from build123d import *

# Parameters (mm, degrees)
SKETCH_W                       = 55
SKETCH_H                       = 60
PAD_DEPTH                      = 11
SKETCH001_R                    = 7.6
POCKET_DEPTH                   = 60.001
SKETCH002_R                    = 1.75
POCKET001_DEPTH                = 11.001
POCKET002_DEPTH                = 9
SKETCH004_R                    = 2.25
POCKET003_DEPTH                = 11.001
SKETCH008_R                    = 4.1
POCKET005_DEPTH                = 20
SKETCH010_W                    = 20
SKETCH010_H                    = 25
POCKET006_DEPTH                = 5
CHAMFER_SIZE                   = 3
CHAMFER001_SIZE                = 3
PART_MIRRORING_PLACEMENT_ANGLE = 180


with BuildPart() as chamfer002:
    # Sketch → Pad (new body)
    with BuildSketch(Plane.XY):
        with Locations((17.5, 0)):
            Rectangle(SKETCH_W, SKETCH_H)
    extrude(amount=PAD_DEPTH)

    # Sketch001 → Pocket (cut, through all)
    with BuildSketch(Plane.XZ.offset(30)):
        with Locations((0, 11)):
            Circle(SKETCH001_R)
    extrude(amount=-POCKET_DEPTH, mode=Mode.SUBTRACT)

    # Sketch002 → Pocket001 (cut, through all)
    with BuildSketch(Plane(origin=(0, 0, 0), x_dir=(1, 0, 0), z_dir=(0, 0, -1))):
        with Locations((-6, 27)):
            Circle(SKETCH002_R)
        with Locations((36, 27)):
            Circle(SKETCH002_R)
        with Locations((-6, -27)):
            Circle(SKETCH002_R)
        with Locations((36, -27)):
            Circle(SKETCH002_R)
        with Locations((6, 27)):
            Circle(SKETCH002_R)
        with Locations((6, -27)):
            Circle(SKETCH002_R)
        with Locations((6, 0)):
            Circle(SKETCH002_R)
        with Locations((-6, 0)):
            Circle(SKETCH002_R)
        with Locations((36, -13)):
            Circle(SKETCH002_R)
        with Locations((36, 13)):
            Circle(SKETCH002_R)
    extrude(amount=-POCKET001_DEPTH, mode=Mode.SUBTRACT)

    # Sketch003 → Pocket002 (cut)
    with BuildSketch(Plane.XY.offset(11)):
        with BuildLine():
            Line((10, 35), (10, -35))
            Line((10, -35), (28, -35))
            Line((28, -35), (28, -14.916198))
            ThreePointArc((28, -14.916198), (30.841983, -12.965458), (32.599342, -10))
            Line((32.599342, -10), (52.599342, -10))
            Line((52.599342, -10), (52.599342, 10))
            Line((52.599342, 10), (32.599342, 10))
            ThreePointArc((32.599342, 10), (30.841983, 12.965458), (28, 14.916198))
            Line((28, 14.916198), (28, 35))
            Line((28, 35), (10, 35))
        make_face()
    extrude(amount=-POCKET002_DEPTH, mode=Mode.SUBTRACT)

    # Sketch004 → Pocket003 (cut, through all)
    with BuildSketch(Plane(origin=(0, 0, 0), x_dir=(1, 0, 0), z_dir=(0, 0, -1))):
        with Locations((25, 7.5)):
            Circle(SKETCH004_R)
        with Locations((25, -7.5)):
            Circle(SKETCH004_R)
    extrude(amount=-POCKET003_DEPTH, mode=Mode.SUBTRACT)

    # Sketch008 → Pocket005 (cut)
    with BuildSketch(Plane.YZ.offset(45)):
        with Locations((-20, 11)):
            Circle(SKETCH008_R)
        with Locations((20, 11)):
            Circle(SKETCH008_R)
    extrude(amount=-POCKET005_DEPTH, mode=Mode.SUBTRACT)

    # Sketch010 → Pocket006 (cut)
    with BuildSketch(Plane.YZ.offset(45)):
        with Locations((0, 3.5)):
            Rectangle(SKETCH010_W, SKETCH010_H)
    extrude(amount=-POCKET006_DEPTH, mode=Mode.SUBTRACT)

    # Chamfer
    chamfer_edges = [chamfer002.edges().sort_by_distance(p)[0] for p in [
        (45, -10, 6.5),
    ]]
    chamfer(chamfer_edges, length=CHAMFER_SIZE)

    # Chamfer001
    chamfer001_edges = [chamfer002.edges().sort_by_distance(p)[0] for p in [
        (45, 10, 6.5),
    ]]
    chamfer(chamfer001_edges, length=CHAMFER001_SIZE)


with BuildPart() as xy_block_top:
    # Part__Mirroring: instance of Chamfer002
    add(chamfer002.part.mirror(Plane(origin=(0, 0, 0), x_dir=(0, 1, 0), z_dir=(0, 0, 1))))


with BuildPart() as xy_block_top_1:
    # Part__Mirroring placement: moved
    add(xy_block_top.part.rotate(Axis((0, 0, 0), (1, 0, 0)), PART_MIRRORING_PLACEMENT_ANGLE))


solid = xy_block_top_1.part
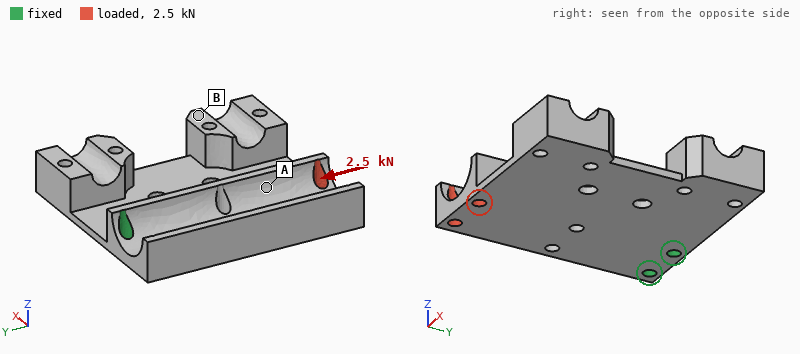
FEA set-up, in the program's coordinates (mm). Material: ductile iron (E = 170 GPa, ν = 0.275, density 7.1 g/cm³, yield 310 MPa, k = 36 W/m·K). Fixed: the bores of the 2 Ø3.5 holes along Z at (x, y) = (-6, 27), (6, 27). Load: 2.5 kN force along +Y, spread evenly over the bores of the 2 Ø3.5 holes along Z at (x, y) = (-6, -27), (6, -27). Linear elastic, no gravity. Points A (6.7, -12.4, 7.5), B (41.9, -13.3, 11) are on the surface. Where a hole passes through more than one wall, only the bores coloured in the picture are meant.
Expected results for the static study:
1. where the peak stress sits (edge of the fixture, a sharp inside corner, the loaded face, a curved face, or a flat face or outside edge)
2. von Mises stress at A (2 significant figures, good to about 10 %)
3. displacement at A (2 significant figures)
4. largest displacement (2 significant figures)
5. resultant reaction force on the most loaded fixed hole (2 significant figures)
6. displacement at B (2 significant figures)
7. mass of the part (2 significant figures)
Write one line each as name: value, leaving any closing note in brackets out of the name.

where the peak stress sits: the loaded face
von Mises stress at A: 18 MPa
displacement at A: 4.8 µm
largest displacement: 9.3 µm
resultant reaction force on the most loaded fixed hole: 1.3 kN
displacement at B: 2.3 µm
mass of the part: 110 g
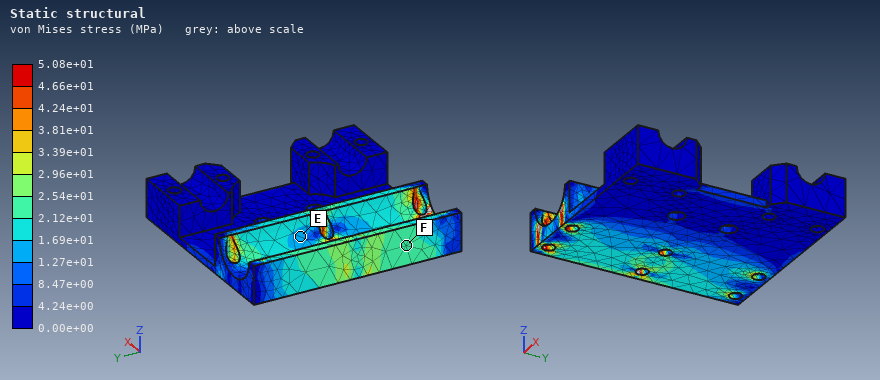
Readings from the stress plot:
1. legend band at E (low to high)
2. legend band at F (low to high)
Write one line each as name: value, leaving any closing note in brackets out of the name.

legend band at E: 1.27e+01 to 1.69e+01 MPa
legend band at F: 2.12e+01 to 2.54e+01 MPa
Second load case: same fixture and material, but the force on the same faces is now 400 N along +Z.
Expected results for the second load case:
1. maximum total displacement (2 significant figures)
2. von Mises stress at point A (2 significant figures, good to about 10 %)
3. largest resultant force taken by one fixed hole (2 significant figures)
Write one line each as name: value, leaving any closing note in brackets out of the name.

maximum total displacement: 0.13 mm
von Mises stress at point A: 26 MPa
largest resultant force taken by one fixed hole: 250 N
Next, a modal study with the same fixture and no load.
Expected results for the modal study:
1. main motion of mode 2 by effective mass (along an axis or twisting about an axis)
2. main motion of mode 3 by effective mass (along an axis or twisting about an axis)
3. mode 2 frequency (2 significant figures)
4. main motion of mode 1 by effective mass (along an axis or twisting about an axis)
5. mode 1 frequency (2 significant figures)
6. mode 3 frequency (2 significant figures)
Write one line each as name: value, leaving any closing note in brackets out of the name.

main motion of mode 2 by effective mass: twisting about X
main motion of mode 3 by effective mass: along Z
mode 2 frequency: 1100 Hz
main motion of mode 1 by effective mass: along Z
mode 1 frequency: 610 Hz
mode 3 frequency: 2200 Hz
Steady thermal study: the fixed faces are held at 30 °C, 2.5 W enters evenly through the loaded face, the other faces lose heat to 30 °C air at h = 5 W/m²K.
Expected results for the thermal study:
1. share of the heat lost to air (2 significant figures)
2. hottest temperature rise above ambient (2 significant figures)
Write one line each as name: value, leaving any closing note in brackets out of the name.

share of the heat lost to air: 20 %
hottest temperature rise above ambient: 23 K
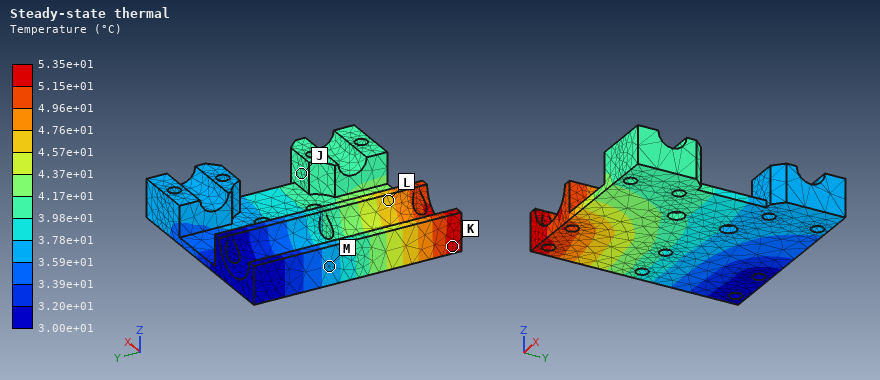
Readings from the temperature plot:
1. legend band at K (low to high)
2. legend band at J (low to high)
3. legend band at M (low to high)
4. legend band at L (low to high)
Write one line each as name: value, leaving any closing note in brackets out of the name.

legend band at K: 5.15e+01 to 5.35e+01 °C
legend band at J: 3.98e+01 to 4.17e+01 °C
legend band at M: 3.59e+01 to 3.78e+01 °C
legend band at L: 4.57e+01 to 4.76e+01 °C
